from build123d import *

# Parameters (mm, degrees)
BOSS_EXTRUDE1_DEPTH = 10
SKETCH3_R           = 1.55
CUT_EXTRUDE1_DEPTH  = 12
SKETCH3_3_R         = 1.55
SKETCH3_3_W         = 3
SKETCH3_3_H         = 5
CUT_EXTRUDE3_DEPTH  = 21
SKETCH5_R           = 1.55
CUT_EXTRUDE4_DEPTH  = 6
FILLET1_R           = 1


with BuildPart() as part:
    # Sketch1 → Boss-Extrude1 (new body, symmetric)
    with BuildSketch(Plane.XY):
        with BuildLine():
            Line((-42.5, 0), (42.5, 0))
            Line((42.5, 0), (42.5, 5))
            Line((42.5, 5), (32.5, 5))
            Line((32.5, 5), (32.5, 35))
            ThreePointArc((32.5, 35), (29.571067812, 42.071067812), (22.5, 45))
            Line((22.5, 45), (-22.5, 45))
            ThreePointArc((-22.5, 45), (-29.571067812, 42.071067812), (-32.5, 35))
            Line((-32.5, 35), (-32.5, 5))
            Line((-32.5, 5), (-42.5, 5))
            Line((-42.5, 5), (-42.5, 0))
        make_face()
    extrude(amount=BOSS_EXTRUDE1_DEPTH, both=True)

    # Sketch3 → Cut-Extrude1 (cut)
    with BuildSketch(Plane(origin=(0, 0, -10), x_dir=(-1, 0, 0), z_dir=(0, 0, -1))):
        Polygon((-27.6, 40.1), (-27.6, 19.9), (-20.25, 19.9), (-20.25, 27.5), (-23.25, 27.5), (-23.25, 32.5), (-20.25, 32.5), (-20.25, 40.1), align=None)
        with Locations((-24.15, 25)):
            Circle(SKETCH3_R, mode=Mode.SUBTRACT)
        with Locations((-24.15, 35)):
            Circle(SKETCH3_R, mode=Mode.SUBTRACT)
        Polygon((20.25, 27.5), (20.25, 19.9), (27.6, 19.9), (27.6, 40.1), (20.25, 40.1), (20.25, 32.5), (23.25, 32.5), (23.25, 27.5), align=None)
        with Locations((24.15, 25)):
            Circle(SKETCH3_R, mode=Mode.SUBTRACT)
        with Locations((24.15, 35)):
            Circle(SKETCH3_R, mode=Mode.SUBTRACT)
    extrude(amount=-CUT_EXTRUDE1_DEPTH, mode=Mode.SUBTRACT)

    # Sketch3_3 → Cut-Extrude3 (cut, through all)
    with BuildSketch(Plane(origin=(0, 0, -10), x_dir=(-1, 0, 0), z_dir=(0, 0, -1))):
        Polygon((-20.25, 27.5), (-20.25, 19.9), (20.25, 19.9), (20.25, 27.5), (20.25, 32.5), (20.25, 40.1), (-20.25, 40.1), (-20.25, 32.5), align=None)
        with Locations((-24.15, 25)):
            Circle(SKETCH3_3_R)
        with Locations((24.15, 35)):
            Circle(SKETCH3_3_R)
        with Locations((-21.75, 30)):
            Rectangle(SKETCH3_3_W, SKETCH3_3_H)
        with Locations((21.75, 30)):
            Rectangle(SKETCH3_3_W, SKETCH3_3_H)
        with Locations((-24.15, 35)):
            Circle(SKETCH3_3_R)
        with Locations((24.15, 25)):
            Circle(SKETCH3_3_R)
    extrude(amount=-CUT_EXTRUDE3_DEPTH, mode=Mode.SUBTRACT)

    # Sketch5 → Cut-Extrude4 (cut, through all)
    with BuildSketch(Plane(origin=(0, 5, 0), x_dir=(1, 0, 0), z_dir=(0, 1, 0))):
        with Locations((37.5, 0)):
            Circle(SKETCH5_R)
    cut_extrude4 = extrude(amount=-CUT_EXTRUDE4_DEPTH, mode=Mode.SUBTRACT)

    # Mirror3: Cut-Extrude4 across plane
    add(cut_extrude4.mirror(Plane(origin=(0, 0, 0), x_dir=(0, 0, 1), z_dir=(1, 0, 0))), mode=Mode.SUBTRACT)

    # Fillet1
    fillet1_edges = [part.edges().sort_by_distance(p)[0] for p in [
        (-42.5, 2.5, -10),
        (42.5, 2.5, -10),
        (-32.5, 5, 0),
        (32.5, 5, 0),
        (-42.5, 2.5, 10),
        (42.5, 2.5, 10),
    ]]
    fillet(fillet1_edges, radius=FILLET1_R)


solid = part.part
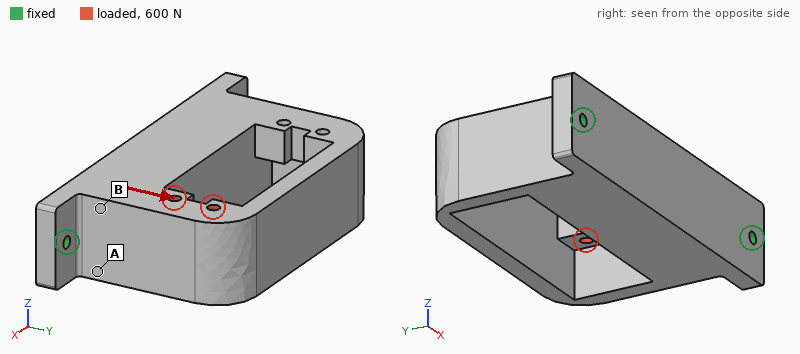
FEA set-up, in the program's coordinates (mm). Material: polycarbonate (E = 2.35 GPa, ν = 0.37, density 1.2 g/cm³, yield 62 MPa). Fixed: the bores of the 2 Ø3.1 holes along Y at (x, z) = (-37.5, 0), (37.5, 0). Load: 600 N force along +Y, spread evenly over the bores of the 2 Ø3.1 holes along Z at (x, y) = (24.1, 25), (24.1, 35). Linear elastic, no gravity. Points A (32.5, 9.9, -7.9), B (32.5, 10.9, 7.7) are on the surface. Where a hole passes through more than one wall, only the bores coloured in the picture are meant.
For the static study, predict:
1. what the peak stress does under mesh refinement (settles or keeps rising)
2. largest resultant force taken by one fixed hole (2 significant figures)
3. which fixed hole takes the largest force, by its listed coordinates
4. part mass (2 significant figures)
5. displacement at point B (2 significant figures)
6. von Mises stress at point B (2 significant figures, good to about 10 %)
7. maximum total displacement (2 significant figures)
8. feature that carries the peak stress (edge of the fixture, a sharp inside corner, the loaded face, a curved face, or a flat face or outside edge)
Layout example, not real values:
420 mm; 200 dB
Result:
keeps rising; 530 N; (37.5, 0); 47 g; 0.35 mm; 8.3 MPa; 1.1 mm; edge of the fixture
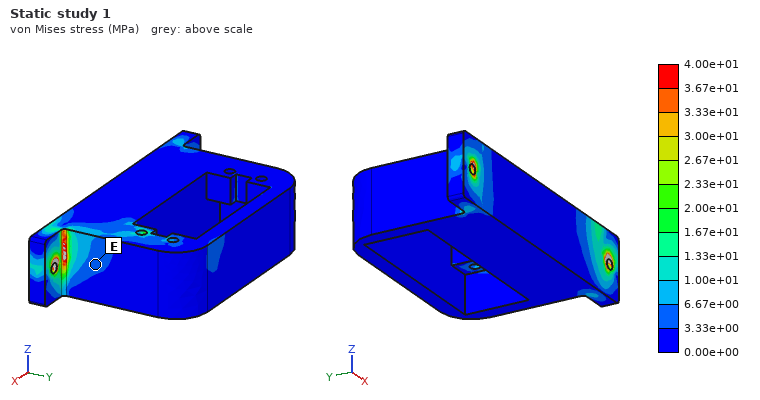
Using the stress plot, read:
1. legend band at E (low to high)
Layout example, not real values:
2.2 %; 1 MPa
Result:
3.33e+00 to 6.67e+00 MPa
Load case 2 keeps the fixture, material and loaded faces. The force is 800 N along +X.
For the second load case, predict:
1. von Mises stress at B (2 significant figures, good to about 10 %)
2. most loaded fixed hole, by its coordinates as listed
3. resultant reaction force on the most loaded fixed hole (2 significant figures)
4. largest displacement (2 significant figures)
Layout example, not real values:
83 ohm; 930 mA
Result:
9.0 MPa; (-37.5, 0); 560 N; 0.53 mm
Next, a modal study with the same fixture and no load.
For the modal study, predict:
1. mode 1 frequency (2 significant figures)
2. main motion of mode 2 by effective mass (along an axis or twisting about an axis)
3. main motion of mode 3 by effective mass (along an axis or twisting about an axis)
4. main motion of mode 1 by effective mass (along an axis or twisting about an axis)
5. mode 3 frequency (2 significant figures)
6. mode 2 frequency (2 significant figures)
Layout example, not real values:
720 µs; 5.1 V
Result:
450 Hz; along X; along Y; along Z; 1800 Hz; 1400 Hz
